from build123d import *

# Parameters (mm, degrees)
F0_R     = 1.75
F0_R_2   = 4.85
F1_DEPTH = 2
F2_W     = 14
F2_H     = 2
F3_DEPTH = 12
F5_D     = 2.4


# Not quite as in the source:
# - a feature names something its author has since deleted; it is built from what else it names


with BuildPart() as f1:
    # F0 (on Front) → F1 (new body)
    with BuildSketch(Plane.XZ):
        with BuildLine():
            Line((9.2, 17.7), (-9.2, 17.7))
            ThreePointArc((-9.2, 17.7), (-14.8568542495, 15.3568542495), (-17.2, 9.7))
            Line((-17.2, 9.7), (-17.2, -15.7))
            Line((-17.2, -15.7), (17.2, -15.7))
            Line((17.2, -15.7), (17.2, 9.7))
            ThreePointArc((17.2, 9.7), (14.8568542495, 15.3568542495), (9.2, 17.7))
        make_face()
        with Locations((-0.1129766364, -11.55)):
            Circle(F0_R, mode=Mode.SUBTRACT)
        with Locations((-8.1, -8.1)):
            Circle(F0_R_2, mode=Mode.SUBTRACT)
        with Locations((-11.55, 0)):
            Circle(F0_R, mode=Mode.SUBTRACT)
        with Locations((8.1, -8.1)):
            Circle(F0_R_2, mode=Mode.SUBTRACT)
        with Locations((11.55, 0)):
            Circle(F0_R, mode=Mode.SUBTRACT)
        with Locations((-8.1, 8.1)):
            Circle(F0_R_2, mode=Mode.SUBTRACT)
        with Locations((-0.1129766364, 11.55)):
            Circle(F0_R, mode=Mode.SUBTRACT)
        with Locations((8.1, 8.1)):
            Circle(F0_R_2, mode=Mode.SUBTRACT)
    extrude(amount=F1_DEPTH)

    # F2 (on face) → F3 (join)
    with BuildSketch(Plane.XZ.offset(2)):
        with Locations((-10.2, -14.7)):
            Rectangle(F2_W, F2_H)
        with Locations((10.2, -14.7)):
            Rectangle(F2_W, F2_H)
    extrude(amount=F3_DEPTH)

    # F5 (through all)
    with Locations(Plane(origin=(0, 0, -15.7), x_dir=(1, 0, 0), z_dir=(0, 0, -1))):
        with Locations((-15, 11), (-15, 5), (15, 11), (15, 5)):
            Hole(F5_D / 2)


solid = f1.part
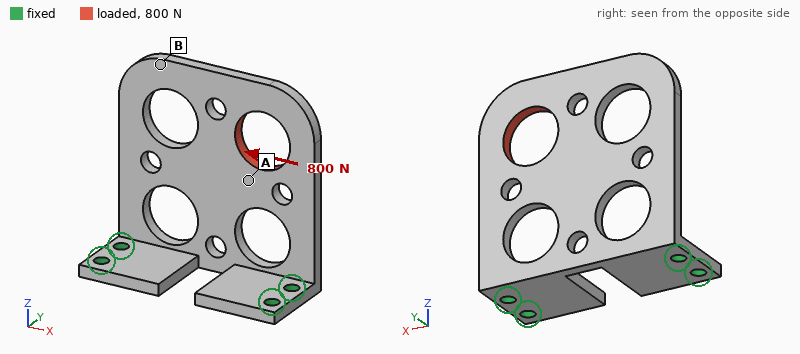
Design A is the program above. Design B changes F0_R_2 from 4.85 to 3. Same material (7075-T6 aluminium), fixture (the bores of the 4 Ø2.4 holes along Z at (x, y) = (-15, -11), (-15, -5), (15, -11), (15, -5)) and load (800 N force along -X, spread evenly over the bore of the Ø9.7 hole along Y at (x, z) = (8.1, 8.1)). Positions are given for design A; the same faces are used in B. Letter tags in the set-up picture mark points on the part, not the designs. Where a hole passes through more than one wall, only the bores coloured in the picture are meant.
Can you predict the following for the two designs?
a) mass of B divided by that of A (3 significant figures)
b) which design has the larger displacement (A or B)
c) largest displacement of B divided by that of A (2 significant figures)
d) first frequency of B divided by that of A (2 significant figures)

1.17
A
0.80
1.1
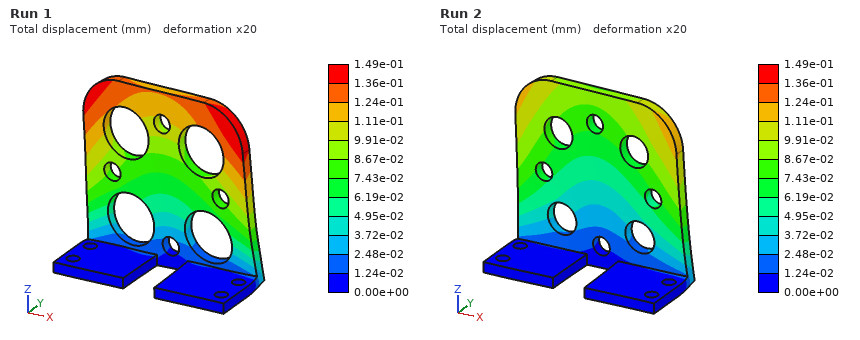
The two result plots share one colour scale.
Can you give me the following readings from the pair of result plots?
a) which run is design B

Run 2
